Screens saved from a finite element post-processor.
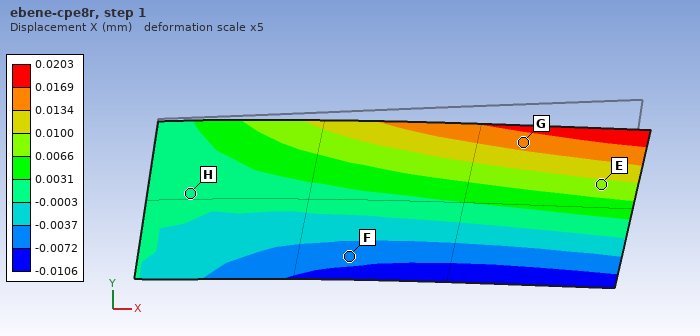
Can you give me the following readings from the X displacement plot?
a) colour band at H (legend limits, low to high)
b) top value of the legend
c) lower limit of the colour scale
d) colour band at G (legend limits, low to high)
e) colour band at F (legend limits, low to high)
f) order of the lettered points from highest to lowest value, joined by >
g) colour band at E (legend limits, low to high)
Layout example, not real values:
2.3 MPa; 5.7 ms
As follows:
-0.0003 to 0.0031 mm; 0.0203 mm; -0.0106 mm; 0.0134 to 0.0169 mm; -0.0072 to -0.0037 mm; G > E > H > F; 0.0066 to 0.0100 mm
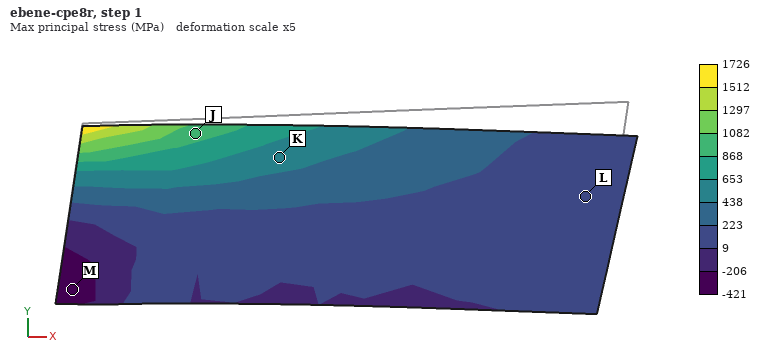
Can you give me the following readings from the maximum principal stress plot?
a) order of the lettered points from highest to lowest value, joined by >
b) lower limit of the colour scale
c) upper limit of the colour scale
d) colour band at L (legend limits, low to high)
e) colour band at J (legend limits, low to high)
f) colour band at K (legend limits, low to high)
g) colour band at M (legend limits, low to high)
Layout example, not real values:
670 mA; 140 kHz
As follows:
J > K > L > M; -421 MPa; 1726 MPa; 9 to 223 MPa; 868 to 1082 MPa; 438 to 653 MPa; -421 to -206 MPa
